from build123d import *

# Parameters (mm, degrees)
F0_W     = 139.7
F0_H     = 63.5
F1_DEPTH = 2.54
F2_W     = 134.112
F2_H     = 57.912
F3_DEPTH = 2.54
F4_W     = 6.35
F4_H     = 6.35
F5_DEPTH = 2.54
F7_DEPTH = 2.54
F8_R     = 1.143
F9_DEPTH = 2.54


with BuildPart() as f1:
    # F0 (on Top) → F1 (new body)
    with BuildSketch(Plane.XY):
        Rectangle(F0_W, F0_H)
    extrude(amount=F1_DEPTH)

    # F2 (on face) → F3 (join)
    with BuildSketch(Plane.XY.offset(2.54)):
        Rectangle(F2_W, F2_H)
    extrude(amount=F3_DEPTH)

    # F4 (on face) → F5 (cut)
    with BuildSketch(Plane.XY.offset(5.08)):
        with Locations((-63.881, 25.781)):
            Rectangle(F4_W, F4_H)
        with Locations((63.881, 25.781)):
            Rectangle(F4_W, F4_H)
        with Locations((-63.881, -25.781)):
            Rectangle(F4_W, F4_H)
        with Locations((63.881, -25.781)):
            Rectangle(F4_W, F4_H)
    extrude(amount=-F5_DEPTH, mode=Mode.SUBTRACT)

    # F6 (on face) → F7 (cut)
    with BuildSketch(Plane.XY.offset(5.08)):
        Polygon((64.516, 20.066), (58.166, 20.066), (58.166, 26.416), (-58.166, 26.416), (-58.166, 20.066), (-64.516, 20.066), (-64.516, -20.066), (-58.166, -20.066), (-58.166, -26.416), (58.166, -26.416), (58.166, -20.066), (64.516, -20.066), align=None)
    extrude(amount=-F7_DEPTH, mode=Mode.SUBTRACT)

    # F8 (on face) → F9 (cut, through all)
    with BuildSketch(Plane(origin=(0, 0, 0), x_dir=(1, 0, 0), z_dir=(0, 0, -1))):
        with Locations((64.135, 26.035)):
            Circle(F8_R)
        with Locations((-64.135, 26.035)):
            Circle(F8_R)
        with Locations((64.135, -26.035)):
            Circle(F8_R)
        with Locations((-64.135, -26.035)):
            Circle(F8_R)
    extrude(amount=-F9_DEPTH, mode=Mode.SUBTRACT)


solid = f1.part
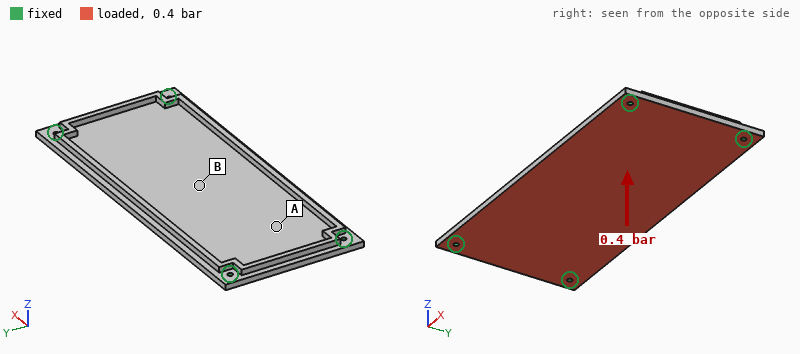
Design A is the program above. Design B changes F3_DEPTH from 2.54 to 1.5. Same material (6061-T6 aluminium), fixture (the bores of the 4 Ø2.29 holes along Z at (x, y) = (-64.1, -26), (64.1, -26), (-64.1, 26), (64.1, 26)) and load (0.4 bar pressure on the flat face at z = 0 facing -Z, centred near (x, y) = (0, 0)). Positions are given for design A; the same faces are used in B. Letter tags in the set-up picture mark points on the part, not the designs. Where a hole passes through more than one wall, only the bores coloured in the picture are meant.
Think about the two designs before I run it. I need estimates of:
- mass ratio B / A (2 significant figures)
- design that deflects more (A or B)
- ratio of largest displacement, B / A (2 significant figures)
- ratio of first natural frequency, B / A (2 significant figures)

0.96
B
1.2
0.91
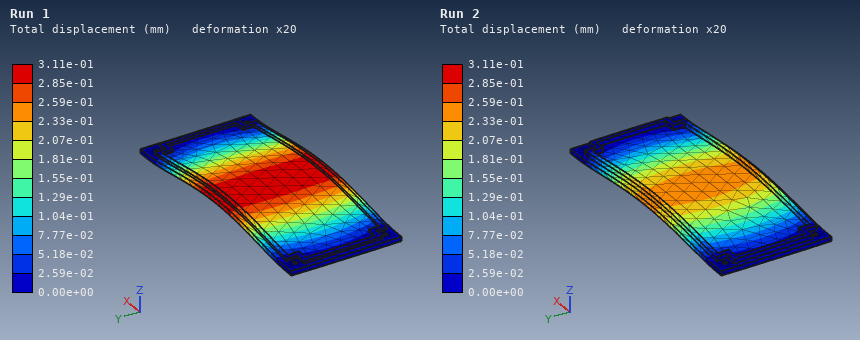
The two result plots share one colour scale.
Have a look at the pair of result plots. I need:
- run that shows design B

Run 1
